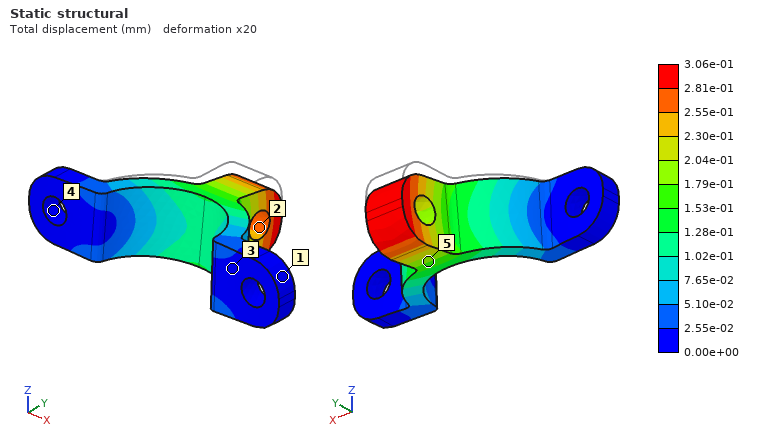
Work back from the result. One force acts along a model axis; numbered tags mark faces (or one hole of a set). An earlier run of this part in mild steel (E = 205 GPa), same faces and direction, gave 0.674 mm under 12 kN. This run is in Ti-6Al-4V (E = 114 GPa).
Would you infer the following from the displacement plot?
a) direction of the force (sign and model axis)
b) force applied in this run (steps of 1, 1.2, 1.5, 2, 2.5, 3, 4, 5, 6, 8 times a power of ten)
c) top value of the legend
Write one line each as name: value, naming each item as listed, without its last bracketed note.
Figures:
direction of the force: -Z
force applied in this run: 3 kN
top value of the legend: 3.06e-01 mm
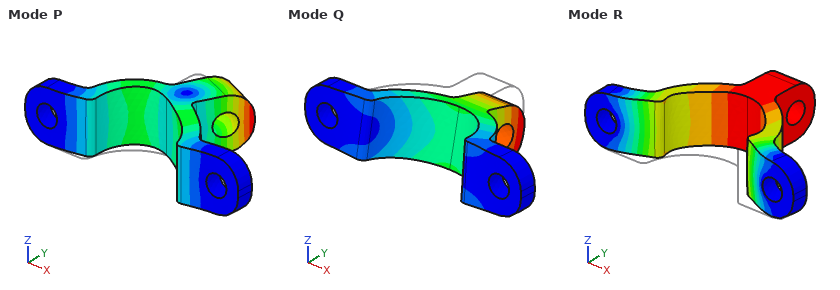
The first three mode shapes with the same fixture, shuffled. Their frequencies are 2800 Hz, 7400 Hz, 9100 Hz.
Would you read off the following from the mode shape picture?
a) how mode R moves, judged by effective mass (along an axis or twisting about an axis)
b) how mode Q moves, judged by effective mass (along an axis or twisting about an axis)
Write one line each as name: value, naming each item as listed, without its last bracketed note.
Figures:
how mode R moves, judged by effective mass: along Y
how mode Q moves, judged by effective mass: along Z
